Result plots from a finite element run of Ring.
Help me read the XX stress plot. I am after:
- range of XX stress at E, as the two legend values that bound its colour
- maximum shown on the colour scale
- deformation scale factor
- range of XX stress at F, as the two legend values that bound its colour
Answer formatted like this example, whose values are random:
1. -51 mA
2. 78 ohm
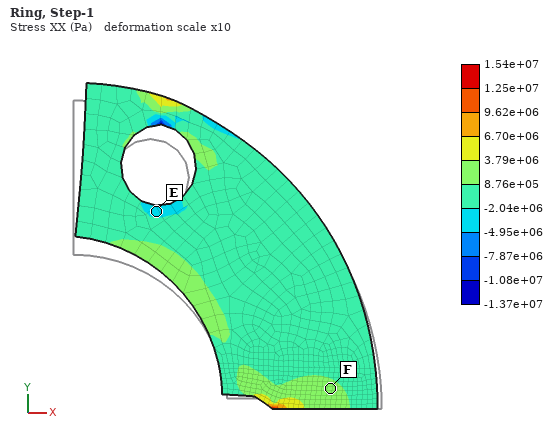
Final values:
1. -4.95e+06 to -2.04e+06 Pa
2. 1.54e+07 Pa
3. 10
4. 8.76e+05 to 3.79e+06 Pa
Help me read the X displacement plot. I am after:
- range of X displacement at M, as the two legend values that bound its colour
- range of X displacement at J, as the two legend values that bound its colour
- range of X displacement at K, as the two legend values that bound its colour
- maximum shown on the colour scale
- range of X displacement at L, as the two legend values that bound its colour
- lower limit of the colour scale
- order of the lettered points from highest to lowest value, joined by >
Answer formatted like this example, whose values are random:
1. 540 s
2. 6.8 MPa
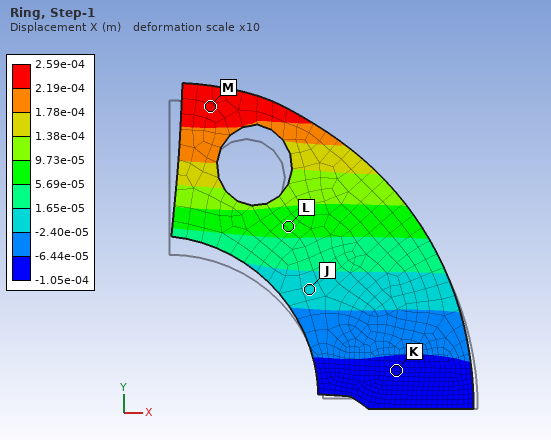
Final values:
1. 2.19e-04 to 2.59e-04 m
2. -2.40e-05 to 1.65e-05 m
3. -1.05e-04 to -6.44e-05 m
4. 2.59e-04 m
5. 5.69e-05 to 9.73e-05 m
6. -1.05e-04 m
7. M > L > J > K
